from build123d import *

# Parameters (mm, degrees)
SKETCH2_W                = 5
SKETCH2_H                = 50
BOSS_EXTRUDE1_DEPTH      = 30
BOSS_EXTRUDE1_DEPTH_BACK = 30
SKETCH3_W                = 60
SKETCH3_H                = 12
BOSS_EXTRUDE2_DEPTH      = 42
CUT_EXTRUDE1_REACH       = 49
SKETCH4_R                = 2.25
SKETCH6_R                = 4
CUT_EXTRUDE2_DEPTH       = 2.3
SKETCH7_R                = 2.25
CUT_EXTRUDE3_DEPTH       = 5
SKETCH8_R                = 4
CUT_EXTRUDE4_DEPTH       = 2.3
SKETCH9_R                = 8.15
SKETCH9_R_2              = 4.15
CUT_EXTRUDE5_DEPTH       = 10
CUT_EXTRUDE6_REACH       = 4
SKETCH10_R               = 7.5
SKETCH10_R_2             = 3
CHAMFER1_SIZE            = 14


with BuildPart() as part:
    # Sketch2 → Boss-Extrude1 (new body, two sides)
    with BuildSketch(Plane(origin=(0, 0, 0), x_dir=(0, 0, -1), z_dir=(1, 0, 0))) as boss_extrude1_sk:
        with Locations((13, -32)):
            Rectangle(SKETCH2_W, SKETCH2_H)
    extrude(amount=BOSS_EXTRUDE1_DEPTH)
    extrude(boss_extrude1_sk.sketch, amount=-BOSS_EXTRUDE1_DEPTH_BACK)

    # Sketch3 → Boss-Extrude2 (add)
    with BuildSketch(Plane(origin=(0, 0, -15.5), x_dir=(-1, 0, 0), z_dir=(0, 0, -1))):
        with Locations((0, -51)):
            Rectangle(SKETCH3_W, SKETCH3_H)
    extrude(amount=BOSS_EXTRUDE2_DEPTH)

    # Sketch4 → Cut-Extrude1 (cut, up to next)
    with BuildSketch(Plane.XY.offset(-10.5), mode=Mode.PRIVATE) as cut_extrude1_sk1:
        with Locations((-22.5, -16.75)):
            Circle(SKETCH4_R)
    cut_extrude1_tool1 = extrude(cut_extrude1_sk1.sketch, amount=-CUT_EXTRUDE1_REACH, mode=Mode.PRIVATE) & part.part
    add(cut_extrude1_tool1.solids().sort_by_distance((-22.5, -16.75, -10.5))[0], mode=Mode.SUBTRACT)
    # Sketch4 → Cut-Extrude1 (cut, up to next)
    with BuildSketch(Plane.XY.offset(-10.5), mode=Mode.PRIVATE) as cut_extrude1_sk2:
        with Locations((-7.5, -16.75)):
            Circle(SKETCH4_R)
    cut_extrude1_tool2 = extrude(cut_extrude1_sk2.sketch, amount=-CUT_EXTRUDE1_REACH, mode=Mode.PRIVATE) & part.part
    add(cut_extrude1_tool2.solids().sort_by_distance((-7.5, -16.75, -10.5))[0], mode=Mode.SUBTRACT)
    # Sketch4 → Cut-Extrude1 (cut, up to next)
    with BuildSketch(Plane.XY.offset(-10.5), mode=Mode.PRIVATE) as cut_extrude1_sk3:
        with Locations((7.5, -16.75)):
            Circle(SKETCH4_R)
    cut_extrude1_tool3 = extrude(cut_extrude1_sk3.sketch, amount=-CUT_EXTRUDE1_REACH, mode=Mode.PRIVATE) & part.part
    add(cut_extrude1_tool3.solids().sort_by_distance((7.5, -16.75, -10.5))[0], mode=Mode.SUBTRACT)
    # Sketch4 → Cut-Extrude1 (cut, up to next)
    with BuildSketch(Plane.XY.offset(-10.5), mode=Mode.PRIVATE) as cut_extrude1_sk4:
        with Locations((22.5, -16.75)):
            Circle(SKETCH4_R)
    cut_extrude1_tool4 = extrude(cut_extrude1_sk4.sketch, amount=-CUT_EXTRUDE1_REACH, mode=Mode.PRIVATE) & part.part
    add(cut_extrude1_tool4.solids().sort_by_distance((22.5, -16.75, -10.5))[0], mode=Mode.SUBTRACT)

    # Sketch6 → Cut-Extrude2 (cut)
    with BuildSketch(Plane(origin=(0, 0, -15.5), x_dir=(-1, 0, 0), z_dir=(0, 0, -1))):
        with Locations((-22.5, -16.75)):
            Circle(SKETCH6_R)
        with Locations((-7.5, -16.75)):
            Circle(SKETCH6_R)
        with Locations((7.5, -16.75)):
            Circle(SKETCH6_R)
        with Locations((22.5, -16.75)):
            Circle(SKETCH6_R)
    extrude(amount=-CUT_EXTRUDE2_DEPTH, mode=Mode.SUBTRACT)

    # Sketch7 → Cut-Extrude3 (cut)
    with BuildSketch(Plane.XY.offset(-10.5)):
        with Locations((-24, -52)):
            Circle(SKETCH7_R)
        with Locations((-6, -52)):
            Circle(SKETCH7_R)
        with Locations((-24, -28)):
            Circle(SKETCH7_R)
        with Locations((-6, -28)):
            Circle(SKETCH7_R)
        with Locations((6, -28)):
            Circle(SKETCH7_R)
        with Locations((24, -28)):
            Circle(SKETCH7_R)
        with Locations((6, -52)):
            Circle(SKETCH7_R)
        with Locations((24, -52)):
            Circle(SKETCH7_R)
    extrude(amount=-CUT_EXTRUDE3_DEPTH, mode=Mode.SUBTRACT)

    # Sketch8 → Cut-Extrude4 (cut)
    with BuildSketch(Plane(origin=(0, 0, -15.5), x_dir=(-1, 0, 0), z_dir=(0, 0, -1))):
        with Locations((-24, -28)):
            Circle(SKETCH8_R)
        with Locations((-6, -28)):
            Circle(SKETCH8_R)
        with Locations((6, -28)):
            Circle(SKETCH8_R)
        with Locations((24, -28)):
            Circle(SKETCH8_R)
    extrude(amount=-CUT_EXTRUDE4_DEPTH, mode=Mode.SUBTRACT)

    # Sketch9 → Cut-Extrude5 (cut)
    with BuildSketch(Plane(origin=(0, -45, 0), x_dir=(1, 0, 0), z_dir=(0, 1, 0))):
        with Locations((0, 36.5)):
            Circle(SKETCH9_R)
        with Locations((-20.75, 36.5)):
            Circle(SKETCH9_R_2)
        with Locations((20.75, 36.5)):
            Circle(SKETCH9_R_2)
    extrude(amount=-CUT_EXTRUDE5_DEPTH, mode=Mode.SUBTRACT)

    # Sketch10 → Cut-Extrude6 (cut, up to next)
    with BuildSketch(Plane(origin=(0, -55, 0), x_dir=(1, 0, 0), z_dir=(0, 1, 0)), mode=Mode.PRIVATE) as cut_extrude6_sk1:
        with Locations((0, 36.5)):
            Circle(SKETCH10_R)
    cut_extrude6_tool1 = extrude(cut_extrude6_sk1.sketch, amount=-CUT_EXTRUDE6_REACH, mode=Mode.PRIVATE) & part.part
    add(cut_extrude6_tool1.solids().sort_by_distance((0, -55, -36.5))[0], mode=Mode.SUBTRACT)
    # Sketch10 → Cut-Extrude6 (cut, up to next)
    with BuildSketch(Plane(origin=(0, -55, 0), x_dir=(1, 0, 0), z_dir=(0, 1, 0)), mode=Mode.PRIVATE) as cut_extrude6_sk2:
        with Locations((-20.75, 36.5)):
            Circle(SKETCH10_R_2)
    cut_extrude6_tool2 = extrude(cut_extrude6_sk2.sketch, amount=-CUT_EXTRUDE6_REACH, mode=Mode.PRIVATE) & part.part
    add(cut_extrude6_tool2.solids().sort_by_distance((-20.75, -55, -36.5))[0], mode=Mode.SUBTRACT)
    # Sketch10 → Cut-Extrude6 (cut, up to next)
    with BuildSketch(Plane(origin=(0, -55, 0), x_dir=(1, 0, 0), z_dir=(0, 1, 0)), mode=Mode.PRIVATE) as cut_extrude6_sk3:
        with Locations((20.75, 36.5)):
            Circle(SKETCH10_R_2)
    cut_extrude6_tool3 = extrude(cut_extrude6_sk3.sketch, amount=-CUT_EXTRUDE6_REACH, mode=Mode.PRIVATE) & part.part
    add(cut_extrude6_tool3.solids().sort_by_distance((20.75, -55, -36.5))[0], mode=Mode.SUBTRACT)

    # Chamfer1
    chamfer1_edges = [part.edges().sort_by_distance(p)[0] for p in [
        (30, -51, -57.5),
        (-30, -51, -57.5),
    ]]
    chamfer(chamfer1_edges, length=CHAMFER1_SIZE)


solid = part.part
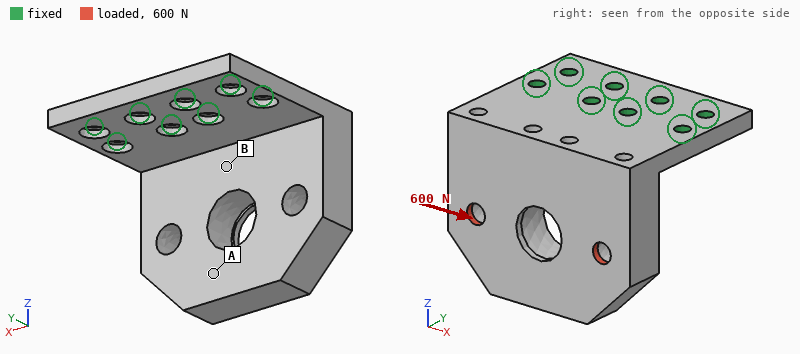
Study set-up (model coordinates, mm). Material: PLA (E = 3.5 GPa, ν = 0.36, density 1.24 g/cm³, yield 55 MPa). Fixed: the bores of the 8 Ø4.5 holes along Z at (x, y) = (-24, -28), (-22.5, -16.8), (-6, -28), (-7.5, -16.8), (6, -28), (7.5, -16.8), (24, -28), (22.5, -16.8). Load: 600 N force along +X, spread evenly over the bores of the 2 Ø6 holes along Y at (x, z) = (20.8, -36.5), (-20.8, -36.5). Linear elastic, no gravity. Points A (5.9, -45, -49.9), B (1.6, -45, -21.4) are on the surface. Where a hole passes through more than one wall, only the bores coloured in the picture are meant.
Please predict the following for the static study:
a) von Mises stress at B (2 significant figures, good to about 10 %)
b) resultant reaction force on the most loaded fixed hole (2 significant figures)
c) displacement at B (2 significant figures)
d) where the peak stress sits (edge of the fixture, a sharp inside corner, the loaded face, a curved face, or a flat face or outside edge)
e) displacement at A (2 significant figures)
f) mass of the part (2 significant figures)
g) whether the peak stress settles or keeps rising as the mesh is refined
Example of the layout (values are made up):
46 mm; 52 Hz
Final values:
7.3 MPa; 510 N; 0.19 mm; edge of the fixture; 0.73 mm; 47 g; keeps rising
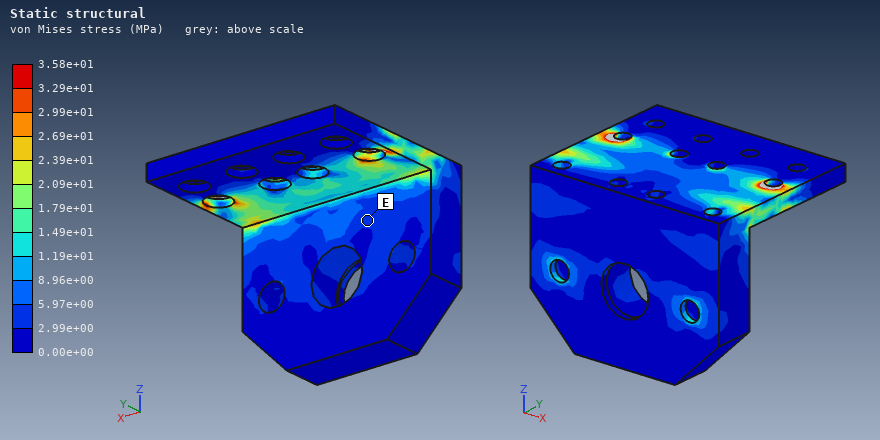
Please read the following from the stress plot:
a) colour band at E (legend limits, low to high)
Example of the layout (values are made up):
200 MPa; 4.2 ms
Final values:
2.99e+00 to 5.97e+00 MPa
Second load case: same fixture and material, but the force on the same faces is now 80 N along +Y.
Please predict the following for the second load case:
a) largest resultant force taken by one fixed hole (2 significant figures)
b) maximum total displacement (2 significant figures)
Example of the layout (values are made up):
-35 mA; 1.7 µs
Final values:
44 N; 0.95 mm
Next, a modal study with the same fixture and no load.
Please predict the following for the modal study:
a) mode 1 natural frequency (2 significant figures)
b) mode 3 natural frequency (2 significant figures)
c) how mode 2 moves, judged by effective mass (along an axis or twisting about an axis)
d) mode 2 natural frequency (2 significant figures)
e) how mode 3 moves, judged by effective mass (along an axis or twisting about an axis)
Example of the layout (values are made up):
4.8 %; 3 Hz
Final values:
300 Hz; 1500 Hz; along X; 780 Hz; along Z
